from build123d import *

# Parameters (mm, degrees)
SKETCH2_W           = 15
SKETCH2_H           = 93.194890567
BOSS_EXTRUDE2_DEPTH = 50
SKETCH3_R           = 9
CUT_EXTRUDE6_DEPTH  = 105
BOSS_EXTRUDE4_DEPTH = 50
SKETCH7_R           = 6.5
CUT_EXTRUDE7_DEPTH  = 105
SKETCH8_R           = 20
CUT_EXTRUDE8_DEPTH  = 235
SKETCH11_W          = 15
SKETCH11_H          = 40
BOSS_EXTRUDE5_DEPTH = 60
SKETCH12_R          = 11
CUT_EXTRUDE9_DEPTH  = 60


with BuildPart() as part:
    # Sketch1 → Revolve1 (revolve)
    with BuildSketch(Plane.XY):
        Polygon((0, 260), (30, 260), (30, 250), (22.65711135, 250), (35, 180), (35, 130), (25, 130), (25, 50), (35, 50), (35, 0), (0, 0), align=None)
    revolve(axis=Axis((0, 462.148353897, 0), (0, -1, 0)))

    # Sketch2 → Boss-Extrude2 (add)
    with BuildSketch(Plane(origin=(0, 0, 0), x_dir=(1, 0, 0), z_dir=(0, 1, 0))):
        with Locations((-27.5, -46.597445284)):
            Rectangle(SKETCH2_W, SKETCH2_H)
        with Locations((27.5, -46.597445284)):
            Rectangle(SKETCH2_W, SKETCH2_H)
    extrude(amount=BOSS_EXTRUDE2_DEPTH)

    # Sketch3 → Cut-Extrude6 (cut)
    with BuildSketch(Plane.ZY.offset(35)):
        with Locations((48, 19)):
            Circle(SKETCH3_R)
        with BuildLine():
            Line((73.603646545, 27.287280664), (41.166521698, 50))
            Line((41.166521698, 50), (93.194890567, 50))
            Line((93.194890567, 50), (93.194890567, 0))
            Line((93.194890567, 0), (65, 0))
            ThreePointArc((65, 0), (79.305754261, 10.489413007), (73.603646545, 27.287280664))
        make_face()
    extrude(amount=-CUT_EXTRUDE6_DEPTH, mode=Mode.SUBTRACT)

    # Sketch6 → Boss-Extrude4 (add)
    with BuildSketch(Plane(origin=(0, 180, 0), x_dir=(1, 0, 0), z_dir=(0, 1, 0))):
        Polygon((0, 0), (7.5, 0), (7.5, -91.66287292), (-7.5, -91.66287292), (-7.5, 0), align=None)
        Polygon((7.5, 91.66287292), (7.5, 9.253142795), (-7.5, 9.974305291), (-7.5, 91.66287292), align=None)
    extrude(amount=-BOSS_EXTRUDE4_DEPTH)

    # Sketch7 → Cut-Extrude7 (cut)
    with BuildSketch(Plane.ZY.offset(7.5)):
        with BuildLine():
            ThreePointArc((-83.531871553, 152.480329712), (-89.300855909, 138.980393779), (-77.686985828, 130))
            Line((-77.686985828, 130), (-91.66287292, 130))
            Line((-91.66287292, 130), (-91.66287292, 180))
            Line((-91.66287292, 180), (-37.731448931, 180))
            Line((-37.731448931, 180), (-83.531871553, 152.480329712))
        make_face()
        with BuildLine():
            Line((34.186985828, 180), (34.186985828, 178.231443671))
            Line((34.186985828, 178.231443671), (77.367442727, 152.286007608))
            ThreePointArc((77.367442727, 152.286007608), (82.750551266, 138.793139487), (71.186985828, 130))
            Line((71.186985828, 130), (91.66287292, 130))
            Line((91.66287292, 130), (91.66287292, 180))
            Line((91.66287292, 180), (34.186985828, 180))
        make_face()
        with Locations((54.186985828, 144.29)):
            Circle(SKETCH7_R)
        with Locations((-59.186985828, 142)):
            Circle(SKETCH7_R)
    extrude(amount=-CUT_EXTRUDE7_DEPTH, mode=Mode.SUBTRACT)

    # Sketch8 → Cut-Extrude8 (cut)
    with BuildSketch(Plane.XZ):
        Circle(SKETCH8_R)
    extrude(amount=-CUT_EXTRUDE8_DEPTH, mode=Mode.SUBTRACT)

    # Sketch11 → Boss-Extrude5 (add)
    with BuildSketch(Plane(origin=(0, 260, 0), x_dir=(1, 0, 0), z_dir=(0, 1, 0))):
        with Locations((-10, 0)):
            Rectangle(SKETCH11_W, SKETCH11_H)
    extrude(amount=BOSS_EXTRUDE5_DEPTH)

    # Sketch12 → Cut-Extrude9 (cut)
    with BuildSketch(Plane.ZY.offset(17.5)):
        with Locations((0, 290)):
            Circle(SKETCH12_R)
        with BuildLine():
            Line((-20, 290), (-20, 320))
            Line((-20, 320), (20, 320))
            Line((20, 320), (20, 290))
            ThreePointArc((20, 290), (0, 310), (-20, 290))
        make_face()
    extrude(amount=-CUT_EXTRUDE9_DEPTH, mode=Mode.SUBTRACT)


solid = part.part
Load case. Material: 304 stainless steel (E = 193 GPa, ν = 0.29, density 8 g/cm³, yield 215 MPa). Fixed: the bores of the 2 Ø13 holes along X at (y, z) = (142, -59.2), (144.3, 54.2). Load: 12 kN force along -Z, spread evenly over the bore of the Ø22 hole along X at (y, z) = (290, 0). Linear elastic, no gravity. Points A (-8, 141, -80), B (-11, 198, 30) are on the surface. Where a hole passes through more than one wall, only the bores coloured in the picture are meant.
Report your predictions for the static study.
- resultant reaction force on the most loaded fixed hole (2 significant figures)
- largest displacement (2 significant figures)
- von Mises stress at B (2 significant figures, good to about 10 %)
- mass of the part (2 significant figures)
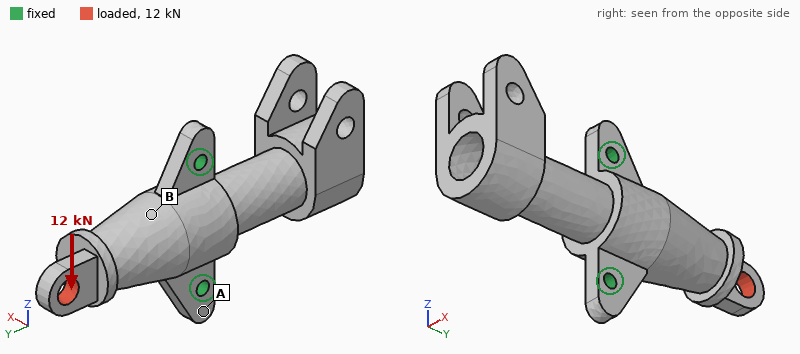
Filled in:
18 kN
0.20 mm
51 MPa
4.8 kg
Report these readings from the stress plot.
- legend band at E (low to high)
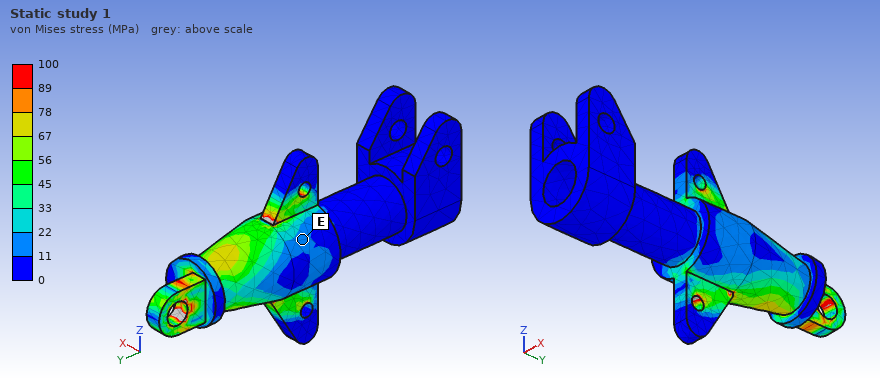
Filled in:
11 to 22 MPa
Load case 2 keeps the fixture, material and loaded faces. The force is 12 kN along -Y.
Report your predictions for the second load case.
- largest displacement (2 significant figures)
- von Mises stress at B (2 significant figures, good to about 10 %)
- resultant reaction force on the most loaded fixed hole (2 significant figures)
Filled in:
89 µm
11 MPa
6.8 kN
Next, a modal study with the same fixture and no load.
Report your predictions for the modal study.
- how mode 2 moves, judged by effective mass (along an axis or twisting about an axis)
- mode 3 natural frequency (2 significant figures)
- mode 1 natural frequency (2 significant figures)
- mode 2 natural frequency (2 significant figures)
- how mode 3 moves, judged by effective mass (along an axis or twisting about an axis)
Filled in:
along Z
1400 Hz
400 Hz
810 Hz
along X
